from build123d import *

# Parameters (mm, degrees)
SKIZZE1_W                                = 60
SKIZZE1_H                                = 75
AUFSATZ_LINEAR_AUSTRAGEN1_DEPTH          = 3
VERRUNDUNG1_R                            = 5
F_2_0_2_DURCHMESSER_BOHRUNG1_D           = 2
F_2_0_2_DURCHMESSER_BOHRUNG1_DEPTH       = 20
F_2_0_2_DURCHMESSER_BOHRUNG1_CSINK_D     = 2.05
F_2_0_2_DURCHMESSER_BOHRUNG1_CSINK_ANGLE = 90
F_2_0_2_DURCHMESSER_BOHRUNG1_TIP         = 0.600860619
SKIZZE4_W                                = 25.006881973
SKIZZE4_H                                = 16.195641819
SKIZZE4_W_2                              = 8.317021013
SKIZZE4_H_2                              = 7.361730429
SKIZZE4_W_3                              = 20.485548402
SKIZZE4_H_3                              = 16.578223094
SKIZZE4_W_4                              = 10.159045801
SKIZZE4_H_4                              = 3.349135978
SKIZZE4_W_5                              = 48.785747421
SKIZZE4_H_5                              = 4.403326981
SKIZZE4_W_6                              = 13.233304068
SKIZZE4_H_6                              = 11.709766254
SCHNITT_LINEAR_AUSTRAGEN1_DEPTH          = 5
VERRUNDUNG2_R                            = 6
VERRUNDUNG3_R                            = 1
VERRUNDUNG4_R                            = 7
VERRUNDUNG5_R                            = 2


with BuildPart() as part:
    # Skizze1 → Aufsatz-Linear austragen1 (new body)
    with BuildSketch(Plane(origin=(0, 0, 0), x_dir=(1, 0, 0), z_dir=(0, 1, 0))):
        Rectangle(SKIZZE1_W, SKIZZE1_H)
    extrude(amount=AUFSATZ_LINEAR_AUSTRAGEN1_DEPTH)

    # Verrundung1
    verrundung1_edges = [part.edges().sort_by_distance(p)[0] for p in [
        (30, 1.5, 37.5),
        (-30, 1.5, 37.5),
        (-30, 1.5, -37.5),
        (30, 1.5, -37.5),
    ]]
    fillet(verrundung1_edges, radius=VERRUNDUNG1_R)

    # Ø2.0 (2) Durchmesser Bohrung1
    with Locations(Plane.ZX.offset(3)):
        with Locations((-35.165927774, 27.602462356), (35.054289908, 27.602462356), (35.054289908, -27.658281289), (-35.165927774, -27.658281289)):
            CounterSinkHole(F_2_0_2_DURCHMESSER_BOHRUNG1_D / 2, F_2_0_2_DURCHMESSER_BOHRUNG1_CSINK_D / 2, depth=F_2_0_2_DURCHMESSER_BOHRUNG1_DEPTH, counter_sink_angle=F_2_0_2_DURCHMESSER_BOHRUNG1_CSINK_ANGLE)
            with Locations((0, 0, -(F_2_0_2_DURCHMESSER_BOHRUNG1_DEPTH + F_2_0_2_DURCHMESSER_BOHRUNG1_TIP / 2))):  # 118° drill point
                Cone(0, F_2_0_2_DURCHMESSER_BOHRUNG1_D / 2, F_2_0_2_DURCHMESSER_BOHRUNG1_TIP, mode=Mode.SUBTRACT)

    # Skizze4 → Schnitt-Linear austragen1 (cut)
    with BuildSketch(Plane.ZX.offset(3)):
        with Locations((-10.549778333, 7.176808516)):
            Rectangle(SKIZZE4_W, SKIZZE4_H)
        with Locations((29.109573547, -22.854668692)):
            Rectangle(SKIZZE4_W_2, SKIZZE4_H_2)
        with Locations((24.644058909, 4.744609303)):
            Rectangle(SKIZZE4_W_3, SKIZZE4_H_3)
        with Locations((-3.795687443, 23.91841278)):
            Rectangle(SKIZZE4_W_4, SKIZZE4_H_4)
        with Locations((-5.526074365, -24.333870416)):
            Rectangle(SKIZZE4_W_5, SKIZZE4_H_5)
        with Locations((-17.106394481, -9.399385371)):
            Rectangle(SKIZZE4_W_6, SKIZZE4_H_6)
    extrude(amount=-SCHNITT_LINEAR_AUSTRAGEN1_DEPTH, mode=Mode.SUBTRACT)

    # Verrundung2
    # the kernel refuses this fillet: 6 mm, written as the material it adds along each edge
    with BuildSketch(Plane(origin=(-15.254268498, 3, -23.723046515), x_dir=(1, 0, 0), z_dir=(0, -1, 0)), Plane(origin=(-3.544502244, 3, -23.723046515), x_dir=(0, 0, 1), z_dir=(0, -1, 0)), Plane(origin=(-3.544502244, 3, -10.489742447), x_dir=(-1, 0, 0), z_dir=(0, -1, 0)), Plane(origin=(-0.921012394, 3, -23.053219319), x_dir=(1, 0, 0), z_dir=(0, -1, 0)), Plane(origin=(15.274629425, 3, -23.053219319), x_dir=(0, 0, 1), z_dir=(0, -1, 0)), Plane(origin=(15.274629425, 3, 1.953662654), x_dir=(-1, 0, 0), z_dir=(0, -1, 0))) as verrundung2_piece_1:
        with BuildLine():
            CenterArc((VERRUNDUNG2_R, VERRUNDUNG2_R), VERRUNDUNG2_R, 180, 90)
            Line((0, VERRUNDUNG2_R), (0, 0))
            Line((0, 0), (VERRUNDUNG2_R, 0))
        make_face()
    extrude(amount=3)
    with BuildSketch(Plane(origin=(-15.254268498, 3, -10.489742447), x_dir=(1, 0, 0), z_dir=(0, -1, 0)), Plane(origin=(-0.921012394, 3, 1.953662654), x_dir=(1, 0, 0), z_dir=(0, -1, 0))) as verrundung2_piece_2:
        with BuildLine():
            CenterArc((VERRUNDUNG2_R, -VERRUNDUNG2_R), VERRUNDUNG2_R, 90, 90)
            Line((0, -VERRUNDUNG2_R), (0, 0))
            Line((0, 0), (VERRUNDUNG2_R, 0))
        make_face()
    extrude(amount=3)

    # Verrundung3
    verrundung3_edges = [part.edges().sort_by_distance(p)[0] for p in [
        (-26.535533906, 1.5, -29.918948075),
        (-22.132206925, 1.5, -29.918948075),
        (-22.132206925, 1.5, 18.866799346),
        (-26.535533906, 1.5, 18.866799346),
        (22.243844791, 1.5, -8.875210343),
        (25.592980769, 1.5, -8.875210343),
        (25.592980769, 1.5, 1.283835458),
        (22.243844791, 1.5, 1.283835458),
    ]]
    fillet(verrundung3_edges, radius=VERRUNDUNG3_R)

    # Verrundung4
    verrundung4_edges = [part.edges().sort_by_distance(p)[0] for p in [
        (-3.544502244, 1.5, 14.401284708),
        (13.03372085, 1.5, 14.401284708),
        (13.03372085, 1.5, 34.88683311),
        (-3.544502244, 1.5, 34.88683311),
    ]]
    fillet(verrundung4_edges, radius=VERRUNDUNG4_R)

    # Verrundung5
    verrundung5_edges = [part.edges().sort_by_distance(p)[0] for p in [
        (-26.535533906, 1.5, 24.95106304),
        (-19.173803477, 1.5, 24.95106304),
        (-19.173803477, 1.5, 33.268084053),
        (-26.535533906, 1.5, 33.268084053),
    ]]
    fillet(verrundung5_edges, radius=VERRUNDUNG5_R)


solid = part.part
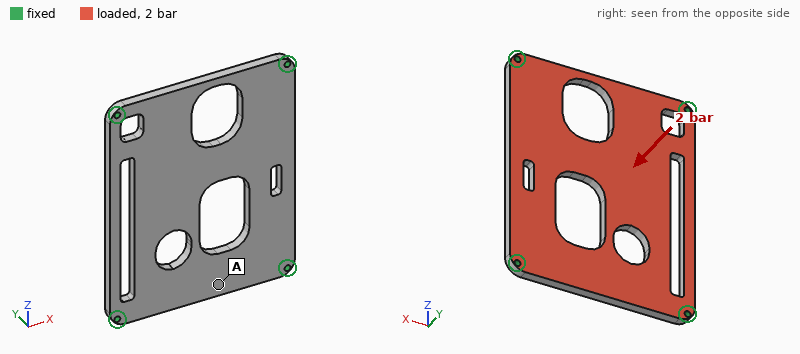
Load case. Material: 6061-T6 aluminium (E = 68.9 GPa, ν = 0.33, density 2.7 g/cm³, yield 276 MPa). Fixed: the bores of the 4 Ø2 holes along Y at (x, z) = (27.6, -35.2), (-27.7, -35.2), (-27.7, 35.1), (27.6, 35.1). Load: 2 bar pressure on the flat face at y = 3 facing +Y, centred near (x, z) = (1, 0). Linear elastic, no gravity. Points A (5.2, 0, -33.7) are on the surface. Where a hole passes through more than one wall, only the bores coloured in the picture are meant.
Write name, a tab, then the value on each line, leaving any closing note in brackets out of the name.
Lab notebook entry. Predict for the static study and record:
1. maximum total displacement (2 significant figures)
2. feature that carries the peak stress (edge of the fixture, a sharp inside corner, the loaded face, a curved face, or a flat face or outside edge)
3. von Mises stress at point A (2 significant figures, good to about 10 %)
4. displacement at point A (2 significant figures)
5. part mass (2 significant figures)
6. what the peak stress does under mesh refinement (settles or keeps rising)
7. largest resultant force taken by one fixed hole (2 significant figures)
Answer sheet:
maximum total displacement	0.23 mm
feature that carries the peak stress	edge of the fixture
von Mises stress at point A	28 MPa
displacement at point A	0.069 mm
part mass	27 g
what the peak stress does under mesh refinement	keeps rising
largest resultant force taken by one fixed hole	180 N
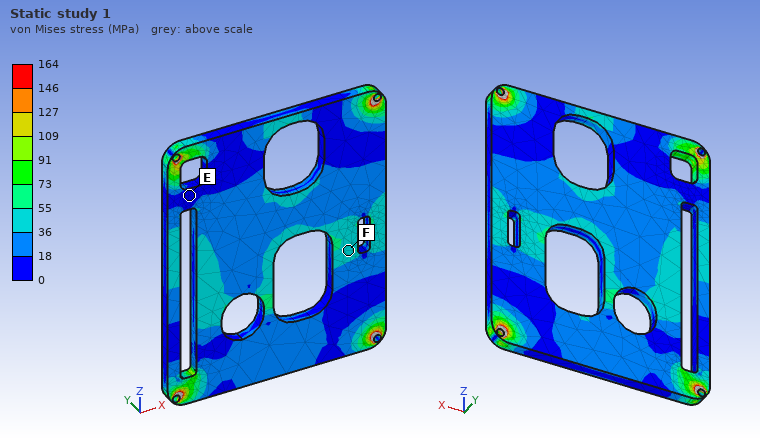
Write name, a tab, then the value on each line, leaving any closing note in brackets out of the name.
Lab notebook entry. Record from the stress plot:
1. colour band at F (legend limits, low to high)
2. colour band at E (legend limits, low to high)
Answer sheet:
colour band at F	36 to 55 MPa
colour band at E	0 to 18 MPa
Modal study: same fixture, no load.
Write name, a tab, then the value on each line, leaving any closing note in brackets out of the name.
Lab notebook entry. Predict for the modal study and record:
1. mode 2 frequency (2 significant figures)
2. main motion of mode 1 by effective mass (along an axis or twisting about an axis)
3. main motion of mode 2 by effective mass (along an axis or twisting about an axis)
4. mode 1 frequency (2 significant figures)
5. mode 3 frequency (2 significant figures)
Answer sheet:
mode 2 frequency	3400 Hz
main motion of mode 1 by effective mass	along Y
main motion of mode 2 by effective mass	twisting about Z
mode 1 frequency	2000 Hz
mode 3 frequency	4200 Hz
